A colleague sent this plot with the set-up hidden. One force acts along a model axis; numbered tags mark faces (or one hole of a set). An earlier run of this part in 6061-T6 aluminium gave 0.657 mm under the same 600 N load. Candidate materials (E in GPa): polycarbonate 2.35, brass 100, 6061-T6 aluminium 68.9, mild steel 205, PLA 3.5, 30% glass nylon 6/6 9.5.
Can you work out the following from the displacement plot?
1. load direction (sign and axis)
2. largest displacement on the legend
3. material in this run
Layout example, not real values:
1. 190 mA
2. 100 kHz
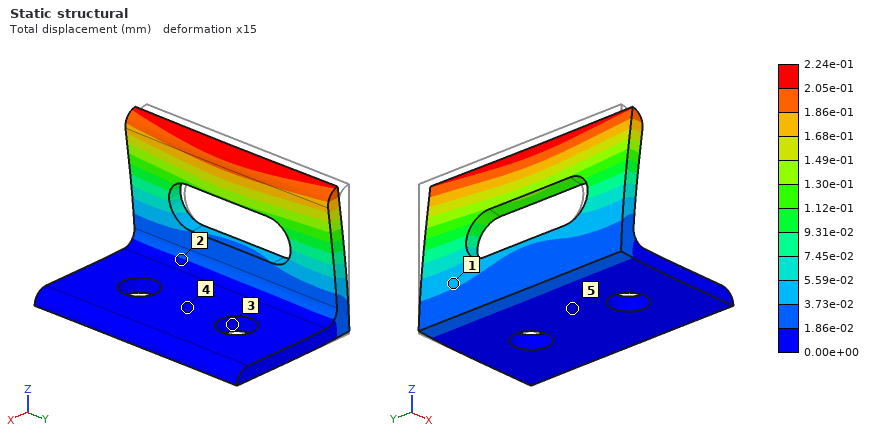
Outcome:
1. +X
2. 2.24e-01 mm
3. mild steel
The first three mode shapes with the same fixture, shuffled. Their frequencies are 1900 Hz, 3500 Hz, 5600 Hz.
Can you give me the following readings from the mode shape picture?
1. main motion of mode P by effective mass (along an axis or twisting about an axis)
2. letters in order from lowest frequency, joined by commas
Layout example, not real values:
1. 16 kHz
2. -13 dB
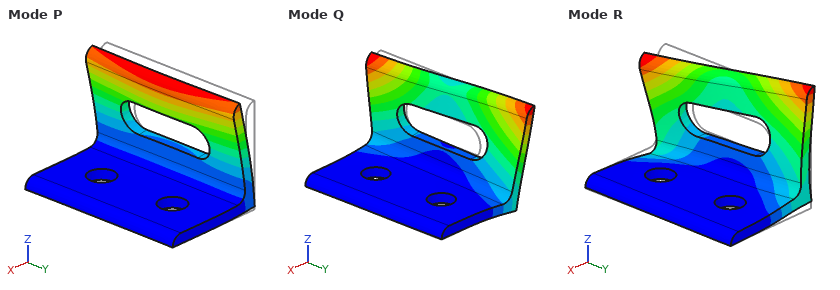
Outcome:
1. along X
2. P, Q, R
